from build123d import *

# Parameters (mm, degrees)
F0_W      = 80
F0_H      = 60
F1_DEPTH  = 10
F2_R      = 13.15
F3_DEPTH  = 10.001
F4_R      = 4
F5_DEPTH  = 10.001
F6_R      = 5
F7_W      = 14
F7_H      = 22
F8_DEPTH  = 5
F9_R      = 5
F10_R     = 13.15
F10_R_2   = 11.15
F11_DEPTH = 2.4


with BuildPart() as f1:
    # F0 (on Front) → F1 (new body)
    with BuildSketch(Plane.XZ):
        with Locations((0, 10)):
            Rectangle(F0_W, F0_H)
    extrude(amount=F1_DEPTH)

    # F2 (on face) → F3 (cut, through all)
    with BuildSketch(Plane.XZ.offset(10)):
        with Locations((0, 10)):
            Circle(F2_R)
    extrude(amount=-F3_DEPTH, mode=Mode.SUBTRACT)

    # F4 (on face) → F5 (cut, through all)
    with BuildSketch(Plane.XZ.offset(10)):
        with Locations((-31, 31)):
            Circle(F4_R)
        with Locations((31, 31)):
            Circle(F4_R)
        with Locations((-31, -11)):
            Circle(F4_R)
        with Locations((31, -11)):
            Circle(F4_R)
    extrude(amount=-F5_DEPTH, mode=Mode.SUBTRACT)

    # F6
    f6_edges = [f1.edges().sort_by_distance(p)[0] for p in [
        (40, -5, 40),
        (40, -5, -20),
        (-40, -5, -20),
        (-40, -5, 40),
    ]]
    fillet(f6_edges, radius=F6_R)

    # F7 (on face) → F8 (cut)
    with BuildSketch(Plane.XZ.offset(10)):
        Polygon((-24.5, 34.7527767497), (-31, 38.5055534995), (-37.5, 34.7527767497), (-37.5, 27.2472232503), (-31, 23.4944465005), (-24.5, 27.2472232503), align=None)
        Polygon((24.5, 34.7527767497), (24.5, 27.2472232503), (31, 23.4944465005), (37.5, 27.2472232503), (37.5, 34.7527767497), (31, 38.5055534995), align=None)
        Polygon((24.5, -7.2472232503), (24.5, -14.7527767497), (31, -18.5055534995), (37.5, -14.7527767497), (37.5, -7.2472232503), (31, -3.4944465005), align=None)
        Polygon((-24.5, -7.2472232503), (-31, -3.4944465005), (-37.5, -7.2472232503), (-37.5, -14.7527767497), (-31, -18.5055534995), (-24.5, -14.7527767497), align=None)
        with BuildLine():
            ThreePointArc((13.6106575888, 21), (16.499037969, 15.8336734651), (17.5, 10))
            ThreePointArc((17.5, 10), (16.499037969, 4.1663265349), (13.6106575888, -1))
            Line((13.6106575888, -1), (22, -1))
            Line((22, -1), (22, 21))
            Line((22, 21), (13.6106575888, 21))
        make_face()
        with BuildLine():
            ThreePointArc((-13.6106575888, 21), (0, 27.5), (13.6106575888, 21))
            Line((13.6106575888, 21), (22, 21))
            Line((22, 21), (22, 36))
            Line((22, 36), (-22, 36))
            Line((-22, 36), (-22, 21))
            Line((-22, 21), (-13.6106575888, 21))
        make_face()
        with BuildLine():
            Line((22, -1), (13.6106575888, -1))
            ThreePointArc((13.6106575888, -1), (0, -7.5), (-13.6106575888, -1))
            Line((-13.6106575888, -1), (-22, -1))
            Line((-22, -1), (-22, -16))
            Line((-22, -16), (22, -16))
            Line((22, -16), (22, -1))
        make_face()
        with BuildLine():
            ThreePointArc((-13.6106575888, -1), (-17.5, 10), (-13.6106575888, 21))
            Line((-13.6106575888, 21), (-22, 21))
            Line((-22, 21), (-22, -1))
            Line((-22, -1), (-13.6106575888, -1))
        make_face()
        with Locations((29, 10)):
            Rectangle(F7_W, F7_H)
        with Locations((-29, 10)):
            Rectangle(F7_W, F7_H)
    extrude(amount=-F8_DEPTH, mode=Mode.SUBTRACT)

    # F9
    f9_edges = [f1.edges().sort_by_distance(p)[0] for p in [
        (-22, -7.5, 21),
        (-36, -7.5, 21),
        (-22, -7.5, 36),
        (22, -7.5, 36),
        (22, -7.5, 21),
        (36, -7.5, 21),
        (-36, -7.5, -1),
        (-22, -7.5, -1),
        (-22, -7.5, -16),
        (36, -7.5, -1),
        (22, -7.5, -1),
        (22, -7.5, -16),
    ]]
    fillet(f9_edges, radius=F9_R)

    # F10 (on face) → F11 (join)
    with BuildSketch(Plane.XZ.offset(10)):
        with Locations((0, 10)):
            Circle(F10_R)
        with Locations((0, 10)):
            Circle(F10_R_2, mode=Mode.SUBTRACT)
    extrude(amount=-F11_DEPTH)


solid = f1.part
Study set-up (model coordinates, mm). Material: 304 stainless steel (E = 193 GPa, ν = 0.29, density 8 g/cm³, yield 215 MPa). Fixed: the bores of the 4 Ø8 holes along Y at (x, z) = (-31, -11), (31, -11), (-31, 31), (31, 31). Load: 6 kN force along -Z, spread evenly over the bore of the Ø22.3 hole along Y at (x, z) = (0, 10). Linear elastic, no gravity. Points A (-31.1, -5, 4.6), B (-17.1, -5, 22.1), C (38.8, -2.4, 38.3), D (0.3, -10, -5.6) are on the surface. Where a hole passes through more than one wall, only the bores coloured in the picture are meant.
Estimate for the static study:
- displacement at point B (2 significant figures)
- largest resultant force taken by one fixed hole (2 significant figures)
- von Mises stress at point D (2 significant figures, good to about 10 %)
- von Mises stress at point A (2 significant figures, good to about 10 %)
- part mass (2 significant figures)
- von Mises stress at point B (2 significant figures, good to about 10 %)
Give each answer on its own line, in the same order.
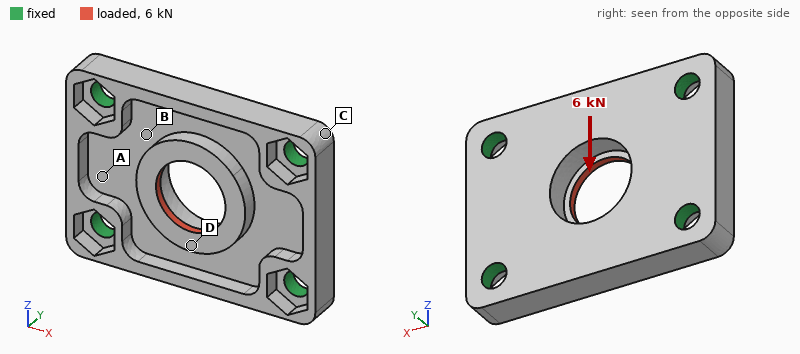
3.8 µm
1.8 kN
42 MPa
16 MPa
230 g
37 MPa
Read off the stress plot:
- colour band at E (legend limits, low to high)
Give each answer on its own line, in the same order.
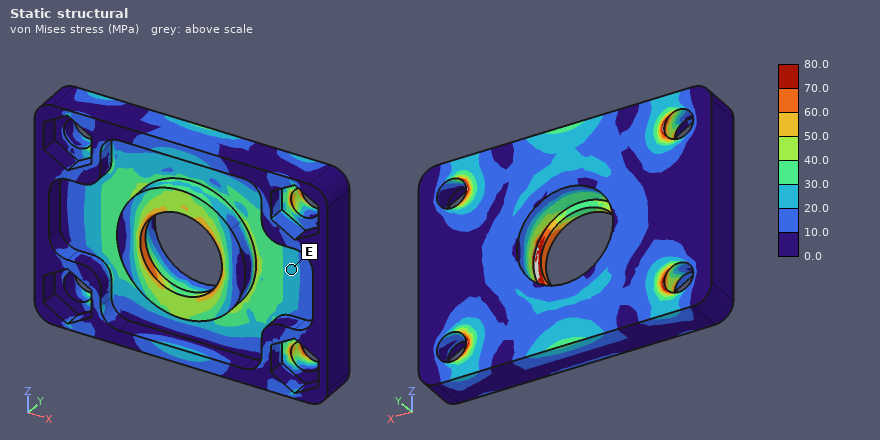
20.0 to 30.0 MPa
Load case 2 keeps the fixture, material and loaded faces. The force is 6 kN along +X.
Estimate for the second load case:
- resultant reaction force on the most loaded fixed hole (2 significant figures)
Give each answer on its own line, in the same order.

1.6 kN
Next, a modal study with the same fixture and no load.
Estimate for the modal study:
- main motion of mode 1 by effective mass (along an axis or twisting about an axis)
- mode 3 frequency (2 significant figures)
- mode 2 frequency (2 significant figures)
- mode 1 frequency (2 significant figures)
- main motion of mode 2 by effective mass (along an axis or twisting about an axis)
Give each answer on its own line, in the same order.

along Y
14 kHz
10 kHz
8700 Hz
twisting about X
